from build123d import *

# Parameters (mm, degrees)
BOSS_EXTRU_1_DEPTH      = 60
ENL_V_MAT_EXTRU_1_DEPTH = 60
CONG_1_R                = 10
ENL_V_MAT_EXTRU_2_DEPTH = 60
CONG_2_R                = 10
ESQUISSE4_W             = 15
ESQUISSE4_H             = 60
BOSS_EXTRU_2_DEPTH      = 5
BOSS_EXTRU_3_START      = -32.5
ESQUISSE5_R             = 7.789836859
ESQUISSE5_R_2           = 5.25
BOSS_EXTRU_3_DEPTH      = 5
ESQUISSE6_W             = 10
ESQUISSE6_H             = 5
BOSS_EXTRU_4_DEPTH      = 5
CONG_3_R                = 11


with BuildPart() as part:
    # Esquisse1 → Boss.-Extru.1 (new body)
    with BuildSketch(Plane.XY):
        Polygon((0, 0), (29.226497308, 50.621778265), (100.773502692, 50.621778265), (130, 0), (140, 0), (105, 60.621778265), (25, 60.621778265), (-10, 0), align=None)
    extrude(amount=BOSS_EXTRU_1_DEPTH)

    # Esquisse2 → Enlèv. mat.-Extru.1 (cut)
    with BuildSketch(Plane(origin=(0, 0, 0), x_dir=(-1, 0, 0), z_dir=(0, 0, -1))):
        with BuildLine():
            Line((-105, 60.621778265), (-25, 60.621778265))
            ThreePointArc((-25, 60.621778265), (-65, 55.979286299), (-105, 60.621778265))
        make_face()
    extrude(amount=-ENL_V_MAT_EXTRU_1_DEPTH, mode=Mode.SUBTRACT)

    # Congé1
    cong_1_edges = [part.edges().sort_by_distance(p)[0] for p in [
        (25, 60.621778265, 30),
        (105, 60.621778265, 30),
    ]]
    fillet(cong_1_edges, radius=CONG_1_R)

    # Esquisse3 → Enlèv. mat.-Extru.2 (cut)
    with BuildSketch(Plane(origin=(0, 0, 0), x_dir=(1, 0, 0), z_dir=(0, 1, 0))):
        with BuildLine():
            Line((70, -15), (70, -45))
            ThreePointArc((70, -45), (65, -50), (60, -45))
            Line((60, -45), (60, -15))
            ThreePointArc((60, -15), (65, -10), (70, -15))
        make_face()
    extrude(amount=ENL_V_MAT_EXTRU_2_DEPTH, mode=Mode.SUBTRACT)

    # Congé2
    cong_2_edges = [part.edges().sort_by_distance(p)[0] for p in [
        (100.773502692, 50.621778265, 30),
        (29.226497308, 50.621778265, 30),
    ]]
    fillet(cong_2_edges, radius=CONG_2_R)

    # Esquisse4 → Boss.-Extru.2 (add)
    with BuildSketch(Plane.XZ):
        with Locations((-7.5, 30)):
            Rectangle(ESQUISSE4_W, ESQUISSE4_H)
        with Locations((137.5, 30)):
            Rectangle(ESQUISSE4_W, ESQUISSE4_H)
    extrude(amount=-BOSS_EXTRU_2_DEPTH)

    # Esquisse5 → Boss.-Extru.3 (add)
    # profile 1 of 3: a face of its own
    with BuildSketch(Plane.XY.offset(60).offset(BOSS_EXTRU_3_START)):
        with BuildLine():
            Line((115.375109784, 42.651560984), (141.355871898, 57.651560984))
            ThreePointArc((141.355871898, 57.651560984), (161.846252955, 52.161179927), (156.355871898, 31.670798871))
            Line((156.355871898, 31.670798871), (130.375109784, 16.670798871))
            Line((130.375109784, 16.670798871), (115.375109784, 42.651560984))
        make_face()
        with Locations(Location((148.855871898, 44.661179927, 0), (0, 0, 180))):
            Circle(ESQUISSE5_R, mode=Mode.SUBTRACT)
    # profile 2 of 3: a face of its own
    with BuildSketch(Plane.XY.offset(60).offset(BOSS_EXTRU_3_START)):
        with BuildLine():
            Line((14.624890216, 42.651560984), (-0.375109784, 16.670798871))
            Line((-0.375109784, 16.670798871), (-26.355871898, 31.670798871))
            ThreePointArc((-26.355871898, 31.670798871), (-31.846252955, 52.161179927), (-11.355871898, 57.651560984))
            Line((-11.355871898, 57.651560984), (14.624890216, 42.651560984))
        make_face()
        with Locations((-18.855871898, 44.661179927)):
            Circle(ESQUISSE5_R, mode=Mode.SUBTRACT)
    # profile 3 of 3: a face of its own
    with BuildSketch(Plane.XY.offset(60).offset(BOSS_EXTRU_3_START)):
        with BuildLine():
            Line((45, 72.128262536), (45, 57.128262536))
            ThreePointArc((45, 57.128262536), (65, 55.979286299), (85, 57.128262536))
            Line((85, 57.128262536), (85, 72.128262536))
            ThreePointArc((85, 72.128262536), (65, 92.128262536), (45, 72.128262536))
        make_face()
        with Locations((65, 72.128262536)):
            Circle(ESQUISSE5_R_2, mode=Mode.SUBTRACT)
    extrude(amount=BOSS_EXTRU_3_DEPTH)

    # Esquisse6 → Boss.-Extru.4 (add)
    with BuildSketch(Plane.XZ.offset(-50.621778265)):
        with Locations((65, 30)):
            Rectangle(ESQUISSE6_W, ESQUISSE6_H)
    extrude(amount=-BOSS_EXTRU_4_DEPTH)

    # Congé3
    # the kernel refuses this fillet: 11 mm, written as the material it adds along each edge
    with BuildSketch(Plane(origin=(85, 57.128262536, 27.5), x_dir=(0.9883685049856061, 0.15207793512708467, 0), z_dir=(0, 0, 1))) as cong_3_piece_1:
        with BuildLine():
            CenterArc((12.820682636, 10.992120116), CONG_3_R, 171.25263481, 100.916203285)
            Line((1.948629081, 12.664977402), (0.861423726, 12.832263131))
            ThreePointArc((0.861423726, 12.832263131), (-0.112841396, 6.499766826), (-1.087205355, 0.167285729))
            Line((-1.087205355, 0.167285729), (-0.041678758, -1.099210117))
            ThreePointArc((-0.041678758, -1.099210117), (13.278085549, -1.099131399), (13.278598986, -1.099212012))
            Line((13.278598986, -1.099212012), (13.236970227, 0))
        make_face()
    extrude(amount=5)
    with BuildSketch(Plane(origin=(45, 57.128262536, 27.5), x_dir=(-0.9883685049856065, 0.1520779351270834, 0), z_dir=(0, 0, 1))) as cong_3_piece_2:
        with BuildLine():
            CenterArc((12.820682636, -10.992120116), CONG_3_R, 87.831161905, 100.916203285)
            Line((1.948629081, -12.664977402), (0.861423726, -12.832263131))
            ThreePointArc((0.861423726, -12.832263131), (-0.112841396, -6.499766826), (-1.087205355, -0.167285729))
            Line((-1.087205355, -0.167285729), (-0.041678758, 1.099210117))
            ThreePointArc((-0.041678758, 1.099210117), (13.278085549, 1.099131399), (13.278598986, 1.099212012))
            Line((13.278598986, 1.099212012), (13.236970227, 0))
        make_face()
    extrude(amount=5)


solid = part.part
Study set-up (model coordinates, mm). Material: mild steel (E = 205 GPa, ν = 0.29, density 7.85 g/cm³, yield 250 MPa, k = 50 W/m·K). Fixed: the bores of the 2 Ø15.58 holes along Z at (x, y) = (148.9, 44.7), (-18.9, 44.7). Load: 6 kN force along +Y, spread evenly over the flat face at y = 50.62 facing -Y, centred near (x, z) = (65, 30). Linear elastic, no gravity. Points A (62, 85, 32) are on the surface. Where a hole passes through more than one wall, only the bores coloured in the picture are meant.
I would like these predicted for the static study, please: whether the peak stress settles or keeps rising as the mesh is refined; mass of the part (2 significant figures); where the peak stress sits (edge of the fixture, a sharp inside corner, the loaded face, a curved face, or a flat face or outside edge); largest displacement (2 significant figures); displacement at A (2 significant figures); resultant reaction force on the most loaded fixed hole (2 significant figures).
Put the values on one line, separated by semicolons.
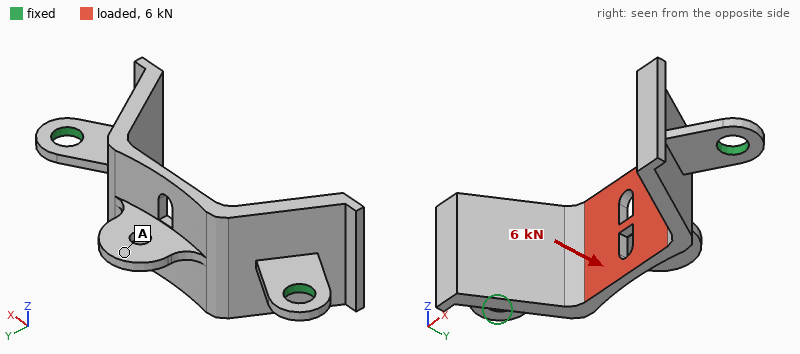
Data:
keeps rising; 910 g; edge of the fixture; 84 µm; 59 µm; 5.0 kN
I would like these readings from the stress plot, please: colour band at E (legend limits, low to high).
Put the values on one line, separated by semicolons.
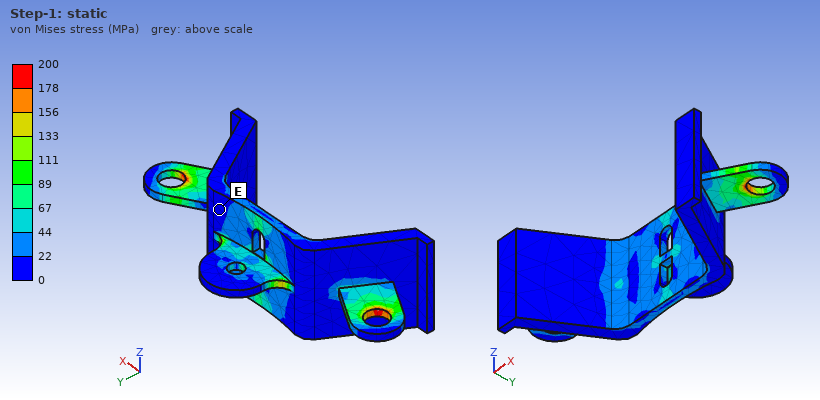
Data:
0 to 22 MPa
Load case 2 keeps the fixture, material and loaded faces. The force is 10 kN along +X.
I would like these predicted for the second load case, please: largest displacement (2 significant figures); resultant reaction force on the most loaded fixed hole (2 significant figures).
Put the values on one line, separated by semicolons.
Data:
35 µm; 5.0 kN
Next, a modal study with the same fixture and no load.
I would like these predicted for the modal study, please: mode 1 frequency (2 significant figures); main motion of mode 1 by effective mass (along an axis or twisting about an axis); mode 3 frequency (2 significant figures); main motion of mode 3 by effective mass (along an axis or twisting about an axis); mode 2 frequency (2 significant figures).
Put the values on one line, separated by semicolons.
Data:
650 Hz; twisting about X; 1400 Hz; along Z; 1300 Hz
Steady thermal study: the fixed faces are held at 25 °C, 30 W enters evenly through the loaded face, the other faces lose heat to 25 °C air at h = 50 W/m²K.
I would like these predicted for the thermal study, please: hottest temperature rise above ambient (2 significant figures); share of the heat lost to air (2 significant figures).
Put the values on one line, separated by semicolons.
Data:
30 K; 80 %
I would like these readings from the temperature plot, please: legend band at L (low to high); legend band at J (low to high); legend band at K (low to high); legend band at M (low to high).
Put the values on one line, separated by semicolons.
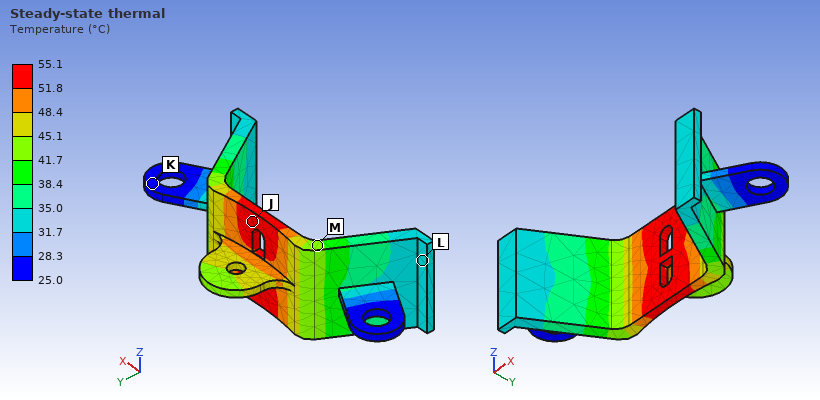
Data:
31.7 to 35.0 °C; 51.8 to 55.1 °C; 25.0 to 28.3 °C; 41.7 to 45.1 °C
